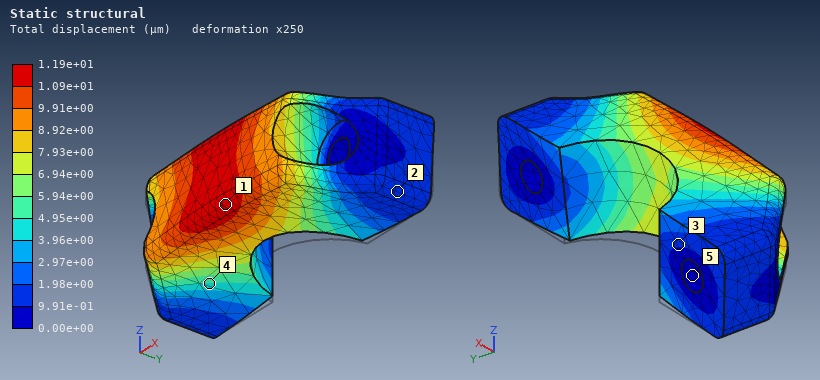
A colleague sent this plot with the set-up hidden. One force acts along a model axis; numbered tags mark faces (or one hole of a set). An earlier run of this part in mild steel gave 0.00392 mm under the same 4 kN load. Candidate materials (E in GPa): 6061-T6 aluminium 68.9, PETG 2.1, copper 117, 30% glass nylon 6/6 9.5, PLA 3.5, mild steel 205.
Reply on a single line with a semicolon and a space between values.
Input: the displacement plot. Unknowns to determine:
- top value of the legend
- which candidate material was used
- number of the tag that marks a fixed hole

1.19e+01 µm; 6061-T6 aluminium; 5
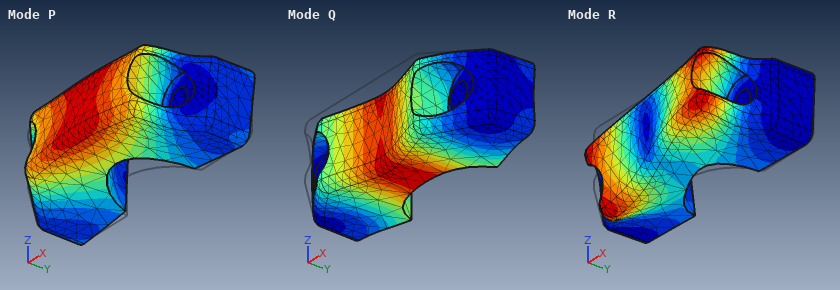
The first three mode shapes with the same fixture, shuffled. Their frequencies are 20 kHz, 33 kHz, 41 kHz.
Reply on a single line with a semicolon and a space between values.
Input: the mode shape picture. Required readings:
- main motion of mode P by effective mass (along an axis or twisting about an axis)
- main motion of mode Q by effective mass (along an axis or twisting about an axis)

along Z; along Y
